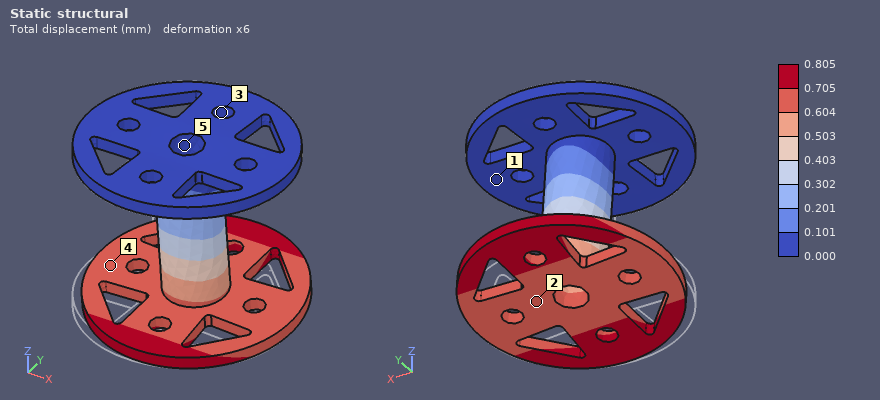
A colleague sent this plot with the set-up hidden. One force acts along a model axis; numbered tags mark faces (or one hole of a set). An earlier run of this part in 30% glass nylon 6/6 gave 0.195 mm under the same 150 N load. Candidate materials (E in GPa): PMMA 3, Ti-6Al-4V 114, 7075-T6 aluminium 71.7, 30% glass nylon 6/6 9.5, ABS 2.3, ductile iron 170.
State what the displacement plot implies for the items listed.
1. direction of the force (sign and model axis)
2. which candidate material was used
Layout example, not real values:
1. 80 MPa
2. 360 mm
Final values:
1. +Y
2. ABS
